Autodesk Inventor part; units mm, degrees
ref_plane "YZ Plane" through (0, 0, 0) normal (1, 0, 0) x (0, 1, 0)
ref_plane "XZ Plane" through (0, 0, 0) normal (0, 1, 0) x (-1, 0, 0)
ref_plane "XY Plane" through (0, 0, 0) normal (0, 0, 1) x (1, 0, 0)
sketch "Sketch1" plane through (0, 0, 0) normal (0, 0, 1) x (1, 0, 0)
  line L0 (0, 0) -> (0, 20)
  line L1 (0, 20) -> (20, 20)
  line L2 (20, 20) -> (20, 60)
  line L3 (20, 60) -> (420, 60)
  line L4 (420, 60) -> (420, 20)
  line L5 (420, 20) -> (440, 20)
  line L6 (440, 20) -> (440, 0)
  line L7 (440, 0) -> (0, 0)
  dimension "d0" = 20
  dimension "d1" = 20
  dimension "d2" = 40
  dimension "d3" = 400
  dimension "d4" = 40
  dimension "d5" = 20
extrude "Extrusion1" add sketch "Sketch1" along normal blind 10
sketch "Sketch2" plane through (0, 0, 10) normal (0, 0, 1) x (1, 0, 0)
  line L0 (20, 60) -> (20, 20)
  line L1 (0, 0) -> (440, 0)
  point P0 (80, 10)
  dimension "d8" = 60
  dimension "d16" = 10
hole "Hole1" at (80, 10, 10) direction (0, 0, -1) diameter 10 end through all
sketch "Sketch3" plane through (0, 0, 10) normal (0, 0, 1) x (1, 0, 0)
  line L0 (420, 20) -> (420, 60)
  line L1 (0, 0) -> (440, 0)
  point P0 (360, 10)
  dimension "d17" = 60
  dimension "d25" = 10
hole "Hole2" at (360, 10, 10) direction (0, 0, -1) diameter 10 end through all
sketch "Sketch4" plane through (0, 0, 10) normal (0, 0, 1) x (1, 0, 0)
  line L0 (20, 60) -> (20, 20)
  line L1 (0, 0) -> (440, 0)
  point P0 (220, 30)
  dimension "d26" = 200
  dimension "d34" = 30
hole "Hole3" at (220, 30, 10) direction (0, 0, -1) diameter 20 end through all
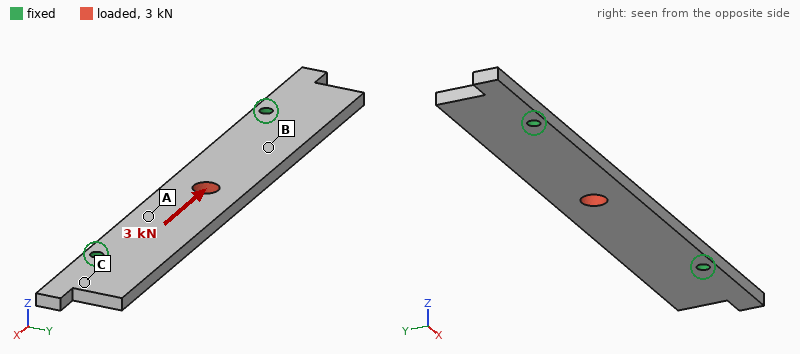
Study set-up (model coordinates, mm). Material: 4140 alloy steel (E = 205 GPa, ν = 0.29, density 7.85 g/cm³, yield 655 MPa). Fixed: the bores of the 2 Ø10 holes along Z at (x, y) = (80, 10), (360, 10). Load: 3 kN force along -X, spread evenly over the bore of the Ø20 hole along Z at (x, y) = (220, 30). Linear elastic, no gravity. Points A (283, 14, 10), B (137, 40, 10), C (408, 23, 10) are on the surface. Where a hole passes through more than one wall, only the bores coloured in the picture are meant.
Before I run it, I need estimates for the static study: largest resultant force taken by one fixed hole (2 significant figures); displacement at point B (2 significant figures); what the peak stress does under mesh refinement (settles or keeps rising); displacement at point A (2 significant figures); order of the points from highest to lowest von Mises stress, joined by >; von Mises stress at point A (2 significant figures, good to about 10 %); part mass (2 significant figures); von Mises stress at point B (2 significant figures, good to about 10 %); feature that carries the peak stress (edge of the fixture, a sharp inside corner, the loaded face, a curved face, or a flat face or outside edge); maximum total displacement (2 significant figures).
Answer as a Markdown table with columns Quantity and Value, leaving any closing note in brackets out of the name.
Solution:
| Quantity | Value |
|---|---|
| largest resultant force taken by one fixed hole | 1.5 kN |
| displacement at point B | 1.7 µm |
| what the peak stress does under mesh refinement | keeps rising |
| displacement at point A | 1.8 µm |
| order of the points from highest to lowest von Mises stress, joined by > | A > B > C |
| von Mises stress at point A | 3.5 MPa |
| part mass | 1.9 kg |
| von Mises stress at point B | 1.9 MPa |
| feature that carries the peak stress | edge of the fixture |
| maximum total displacement | 2.7 µm |
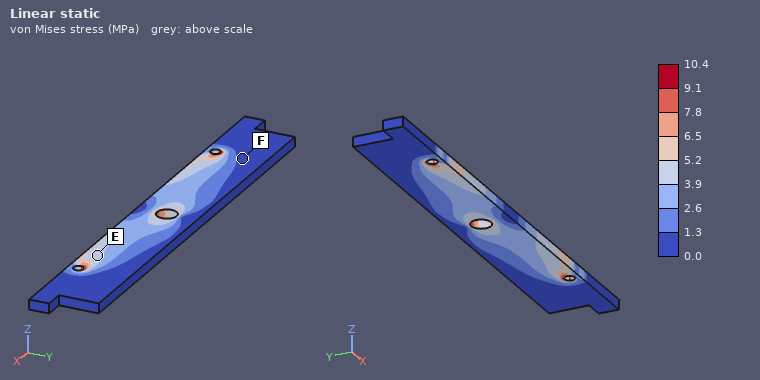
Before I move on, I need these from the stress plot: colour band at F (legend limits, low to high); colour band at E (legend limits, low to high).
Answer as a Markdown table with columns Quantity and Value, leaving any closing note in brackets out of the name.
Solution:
| Quantity | Value |
|---|---|
| colour band at F | 0.0 to 1.3 MPa |
| colour band at E | 3.9 to 5.2 MPa |
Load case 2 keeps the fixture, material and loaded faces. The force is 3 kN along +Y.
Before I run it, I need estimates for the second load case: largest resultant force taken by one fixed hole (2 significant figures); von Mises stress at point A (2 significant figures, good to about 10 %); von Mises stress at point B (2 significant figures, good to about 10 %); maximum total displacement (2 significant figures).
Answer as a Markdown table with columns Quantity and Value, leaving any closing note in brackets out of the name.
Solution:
| Quantity | Value |
|---|---|
| largest resultant force taken by one fixed hole | 2.6 kN |
| von Mises stress at point A | 4.6 MPa |
| von Mises stress at point B | 7.3 MPa |
| maximum total displacement | 23 µm |
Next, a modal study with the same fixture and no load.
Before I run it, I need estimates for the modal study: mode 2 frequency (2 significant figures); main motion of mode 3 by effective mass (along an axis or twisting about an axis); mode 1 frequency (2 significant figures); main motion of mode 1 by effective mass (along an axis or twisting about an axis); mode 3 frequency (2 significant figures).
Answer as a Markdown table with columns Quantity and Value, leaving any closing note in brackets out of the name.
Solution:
| Quantity | Value |
|---|---|
| mode 2 frequency | 1400 Hz |
| main motion of mode 3 by effective mass | along Z |
| mode 1 frequency | 600 Hz |
| main motion of mode 1 by effective mass | along Z |
| mode 3 frequency | 1500 Hz |
